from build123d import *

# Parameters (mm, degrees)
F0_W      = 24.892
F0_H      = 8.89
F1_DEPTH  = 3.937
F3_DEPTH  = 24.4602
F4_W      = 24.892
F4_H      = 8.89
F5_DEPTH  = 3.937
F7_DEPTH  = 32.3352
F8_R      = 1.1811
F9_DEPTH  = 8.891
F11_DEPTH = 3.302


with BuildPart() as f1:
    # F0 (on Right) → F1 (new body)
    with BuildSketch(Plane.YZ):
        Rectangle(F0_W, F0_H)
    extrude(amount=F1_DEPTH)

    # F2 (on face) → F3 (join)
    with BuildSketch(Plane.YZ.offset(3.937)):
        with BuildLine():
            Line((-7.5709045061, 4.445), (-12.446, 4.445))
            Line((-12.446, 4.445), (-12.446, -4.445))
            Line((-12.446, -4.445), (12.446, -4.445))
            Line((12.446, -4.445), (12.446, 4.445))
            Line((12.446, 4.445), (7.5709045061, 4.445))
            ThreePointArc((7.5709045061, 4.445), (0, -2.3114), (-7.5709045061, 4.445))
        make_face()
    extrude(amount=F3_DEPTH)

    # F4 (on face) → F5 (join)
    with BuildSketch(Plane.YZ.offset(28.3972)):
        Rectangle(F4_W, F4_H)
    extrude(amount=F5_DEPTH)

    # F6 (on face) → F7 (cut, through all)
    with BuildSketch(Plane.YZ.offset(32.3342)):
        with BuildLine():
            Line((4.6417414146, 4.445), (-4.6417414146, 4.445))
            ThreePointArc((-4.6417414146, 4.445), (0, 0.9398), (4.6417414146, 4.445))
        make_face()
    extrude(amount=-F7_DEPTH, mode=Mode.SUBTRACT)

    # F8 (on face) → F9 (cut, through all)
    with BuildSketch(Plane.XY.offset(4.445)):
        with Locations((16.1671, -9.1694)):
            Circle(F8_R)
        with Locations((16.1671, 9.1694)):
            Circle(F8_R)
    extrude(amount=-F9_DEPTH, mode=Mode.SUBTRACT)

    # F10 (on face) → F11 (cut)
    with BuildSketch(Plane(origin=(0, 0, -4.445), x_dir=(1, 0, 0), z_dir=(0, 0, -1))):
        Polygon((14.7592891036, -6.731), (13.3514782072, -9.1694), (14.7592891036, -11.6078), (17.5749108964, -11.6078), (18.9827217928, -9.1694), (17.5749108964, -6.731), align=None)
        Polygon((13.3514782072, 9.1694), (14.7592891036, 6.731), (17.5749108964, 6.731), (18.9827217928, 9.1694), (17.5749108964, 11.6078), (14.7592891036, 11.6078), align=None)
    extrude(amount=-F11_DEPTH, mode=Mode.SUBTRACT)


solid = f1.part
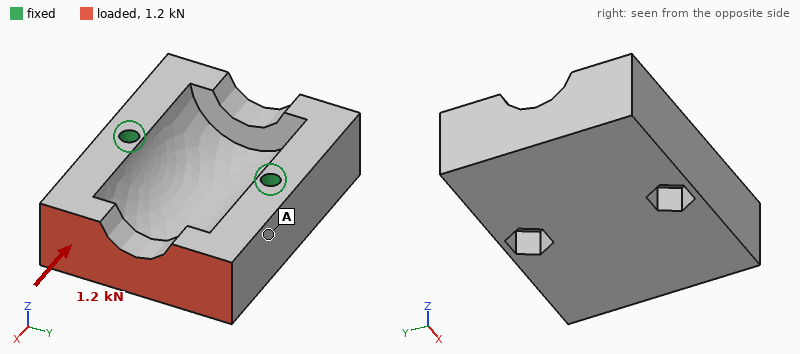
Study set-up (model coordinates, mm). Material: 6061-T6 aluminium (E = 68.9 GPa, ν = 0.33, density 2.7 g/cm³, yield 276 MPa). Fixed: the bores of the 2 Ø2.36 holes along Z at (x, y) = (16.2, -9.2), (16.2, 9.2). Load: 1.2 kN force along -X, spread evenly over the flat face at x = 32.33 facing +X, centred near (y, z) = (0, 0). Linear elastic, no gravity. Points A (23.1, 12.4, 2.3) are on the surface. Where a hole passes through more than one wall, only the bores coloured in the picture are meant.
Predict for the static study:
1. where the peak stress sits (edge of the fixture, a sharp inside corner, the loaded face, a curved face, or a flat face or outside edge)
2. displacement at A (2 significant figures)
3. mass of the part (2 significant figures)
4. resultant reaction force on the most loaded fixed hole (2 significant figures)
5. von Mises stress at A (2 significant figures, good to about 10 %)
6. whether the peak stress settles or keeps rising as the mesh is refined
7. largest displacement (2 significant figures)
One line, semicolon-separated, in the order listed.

edge of the fixture; 2.0 µm; 13 g; 600 N; 8.8 MPa; keeps rising; 5.9 µm
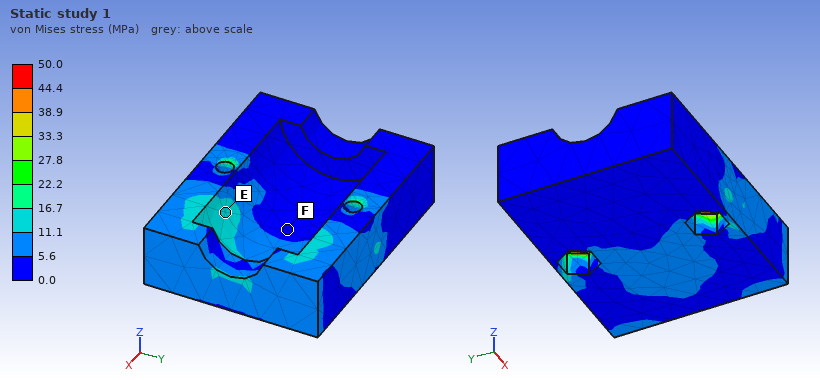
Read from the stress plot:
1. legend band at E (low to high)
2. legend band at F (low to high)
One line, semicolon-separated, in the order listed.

11.1 to 16.7 MPa; 0.0 to 5.6 MPa
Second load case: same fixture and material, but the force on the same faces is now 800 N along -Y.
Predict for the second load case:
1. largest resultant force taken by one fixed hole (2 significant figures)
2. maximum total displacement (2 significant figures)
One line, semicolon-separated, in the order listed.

710 N; 21 µm
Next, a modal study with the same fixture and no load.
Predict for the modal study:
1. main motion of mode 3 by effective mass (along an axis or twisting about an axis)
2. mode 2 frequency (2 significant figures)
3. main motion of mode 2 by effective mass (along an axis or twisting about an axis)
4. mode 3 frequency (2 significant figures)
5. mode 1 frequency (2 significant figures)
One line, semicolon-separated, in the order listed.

along Z; 17 kHz; twisting about Z; 18 kHz; 11 kHz
